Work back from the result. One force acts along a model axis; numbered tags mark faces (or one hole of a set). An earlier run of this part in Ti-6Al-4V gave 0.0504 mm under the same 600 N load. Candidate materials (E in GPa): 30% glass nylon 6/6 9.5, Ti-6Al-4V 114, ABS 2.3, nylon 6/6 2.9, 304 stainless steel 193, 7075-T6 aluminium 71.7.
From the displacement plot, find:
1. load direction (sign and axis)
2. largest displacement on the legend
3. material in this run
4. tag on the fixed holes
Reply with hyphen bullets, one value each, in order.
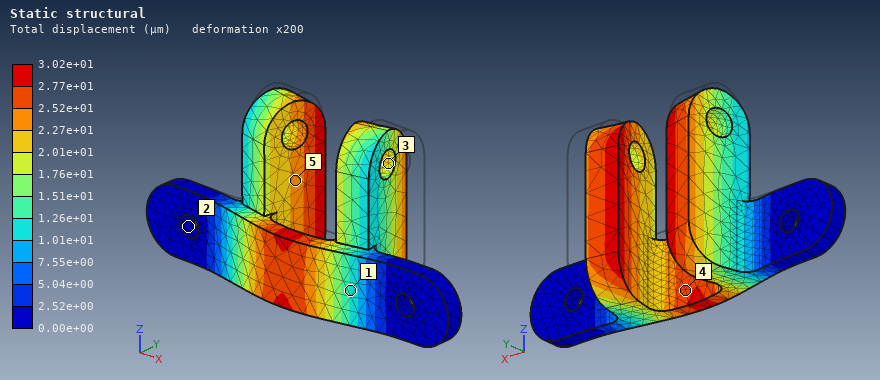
- -Y
- 3.02e+01 µm
- 304 stainless steel
- 2
